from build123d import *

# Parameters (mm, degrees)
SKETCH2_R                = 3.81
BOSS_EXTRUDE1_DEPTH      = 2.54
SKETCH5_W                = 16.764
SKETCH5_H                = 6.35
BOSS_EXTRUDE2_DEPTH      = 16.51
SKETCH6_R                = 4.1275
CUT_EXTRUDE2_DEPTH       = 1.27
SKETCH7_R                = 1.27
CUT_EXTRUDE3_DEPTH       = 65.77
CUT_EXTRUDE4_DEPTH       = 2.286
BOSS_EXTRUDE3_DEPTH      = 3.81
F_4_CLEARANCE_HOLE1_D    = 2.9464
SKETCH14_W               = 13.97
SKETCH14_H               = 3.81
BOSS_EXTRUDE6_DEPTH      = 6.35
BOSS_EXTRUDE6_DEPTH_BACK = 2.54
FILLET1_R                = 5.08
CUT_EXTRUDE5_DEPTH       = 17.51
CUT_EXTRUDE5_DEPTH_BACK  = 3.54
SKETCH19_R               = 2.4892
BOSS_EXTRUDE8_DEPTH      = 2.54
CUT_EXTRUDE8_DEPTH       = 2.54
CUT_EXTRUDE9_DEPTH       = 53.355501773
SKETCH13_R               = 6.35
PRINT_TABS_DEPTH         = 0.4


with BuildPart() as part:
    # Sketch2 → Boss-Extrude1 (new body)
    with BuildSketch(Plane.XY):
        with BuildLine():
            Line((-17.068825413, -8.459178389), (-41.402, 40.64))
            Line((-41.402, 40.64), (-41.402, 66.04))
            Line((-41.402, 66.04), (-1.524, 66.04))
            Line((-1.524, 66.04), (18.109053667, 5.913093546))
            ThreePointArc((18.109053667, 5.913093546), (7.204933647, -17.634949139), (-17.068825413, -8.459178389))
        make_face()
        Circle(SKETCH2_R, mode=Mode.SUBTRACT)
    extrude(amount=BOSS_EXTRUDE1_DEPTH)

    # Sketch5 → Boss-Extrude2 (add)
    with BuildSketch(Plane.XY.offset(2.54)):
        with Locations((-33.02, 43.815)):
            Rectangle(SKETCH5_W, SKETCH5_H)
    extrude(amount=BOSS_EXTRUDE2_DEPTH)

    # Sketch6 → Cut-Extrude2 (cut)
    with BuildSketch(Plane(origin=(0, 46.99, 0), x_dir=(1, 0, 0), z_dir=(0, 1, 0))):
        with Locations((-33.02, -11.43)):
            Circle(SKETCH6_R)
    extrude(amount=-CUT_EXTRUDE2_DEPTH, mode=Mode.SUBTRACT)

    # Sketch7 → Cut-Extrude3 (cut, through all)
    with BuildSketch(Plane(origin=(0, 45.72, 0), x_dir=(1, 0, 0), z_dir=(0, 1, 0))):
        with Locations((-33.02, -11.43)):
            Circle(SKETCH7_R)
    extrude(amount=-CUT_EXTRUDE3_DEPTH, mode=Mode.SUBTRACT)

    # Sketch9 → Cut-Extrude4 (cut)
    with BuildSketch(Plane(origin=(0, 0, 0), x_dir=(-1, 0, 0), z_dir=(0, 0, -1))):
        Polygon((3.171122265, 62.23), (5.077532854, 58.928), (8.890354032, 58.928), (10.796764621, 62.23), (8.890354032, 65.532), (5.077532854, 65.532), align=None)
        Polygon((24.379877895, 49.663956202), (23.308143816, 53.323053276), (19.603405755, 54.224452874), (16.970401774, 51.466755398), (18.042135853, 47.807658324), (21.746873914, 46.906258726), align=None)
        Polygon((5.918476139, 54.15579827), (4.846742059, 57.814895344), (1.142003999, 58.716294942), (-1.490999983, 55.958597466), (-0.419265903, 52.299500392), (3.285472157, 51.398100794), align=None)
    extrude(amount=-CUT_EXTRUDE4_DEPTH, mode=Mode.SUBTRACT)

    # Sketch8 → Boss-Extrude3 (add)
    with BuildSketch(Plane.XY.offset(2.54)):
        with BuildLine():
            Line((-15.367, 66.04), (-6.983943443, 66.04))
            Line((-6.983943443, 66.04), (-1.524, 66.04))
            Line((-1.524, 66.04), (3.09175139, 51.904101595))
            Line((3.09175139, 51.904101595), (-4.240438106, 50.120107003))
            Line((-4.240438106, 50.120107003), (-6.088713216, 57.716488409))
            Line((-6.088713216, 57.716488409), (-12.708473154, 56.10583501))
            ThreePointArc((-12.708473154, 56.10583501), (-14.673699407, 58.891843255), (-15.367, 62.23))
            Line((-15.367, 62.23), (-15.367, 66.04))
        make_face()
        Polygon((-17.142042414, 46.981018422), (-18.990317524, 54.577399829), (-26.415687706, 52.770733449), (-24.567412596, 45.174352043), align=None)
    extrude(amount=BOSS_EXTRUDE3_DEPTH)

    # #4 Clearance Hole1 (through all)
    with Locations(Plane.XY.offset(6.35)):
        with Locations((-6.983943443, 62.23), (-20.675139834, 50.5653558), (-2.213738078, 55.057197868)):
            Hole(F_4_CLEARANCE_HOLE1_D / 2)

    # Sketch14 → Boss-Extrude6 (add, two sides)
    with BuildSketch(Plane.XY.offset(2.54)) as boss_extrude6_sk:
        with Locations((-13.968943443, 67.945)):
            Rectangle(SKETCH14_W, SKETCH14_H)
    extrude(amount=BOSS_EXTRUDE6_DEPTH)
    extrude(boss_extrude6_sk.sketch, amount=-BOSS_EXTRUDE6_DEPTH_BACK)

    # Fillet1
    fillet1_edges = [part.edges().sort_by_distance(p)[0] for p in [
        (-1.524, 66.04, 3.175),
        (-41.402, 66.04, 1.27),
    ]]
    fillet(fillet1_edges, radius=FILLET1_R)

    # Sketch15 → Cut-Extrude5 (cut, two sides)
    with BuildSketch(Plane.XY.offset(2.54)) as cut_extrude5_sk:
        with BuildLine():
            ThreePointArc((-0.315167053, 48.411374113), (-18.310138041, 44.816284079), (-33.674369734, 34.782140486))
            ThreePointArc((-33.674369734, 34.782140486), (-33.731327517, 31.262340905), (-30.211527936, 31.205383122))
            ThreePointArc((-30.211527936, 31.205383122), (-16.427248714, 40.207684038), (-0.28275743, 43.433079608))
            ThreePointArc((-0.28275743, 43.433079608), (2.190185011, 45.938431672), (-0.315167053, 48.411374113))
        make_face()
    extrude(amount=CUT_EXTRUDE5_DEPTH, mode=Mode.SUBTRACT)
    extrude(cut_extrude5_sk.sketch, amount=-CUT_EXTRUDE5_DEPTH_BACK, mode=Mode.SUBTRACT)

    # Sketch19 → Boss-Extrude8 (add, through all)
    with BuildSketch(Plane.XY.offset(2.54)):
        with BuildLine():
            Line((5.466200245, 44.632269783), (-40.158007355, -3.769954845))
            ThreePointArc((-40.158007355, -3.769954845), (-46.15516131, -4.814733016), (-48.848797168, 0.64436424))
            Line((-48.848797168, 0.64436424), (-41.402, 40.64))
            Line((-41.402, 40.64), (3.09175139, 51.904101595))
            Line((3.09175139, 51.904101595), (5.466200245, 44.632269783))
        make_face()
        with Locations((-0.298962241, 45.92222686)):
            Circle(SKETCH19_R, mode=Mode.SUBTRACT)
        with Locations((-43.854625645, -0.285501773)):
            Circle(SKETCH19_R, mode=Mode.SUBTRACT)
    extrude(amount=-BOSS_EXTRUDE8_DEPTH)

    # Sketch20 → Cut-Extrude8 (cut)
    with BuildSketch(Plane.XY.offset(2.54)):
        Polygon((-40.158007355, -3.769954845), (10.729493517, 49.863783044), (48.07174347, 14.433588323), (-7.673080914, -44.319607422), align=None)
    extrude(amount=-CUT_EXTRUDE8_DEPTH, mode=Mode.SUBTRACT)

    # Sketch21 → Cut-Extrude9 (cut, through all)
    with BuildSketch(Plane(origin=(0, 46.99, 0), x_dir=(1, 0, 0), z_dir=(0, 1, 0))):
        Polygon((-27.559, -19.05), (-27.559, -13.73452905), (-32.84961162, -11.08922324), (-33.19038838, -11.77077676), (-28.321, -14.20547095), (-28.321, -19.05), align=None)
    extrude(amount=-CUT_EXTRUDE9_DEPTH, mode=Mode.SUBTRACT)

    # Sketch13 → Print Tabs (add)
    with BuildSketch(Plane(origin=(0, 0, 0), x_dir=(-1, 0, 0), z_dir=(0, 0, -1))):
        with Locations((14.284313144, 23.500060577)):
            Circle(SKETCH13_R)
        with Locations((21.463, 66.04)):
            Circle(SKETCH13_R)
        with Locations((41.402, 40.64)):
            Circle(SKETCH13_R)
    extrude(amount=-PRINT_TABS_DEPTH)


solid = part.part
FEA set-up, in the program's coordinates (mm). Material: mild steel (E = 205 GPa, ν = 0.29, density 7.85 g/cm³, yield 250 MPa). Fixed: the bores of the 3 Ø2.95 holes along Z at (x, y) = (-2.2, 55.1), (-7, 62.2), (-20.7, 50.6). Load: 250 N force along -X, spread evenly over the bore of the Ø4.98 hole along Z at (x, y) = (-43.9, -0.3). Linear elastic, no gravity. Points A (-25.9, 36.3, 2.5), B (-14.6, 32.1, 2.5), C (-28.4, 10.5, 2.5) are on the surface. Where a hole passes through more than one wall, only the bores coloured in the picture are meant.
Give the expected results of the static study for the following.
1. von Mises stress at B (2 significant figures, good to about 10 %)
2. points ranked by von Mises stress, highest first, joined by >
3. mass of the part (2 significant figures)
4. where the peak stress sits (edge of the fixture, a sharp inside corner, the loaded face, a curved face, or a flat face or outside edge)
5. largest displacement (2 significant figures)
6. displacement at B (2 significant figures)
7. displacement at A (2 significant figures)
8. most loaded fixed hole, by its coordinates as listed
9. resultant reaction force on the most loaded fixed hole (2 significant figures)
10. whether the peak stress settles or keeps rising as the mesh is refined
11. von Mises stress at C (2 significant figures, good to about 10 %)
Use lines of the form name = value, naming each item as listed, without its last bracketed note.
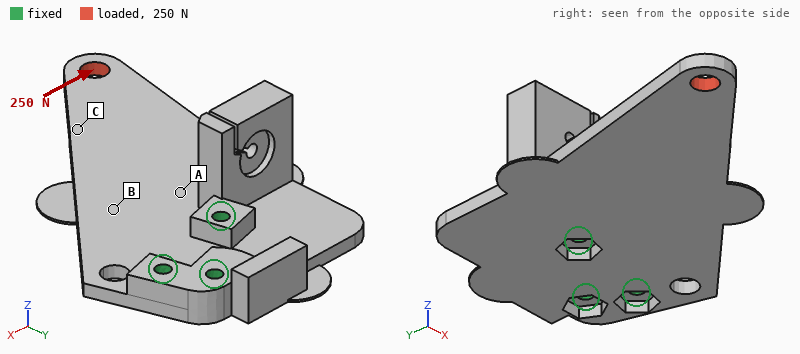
von Mises stress at B = 13 MPa
points ranked by von Mises stress, highest first, joined by > = C > B > A
mass of the part = 66 g
where the peak stress sits = edge of the fixture
largest displacement = 27 µm
displacement at B = 5.4 µm
displacement at A = 4.4 µm
most loaded fixed hole, by its coordinates as listed = (-20.7, 50.6)
resultant reaction force on the most loaded fixed hole = 580 N
whether the peak stress settles or keeps rising as the mesh is refined = keeps rising
von Mises stress at C = 22 MPa
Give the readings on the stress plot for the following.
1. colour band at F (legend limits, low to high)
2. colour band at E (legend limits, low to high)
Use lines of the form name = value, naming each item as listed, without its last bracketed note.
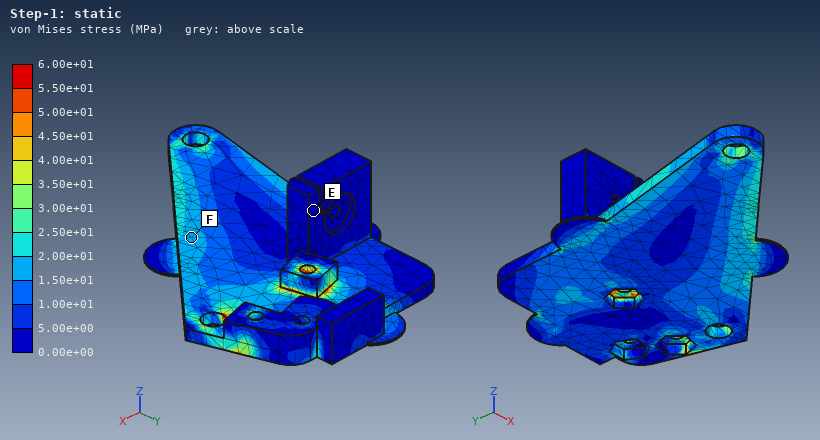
colour band at F = 1.50e+01 to 2.00e+01 MPa
colour band at E = 0.00e+00 to 5.00e+00 MPa
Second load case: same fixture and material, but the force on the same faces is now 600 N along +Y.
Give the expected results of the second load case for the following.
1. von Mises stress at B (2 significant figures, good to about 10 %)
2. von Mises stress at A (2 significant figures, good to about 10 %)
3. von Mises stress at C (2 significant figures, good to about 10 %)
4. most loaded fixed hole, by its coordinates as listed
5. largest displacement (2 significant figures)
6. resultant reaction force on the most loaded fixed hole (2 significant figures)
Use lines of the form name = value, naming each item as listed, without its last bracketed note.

von Mises stress at B = 10 MPa
von Mises stress at A = 9.3 MPa
von Mises stress at C = 14 MPa
most loaded fixed hole, by its coordinates as listed = (-20.7, 50.6)
largest displacement = 42 µm
resultant reaction force on the most loaded fixed hole = 970 N
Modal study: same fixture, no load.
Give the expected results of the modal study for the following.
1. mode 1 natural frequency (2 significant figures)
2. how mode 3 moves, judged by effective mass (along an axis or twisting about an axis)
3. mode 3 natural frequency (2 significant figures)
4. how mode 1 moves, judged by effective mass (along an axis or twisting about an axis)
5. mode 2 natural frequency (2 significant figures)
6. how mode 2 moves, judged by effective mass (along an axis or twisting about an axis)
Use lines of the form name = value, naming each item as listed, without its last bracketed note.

mode 1 natural frequency = 1100 Hz
how mode 3 moves, judged by effective mass = along Z
mode 3 natural frequency = 4100 Hz
how mode 1 moves, judged by effective mass = along Z
mode 2 natural frequency = 3600 Hz
how mode 2 moves, judged by effective mass = twisting about Y
